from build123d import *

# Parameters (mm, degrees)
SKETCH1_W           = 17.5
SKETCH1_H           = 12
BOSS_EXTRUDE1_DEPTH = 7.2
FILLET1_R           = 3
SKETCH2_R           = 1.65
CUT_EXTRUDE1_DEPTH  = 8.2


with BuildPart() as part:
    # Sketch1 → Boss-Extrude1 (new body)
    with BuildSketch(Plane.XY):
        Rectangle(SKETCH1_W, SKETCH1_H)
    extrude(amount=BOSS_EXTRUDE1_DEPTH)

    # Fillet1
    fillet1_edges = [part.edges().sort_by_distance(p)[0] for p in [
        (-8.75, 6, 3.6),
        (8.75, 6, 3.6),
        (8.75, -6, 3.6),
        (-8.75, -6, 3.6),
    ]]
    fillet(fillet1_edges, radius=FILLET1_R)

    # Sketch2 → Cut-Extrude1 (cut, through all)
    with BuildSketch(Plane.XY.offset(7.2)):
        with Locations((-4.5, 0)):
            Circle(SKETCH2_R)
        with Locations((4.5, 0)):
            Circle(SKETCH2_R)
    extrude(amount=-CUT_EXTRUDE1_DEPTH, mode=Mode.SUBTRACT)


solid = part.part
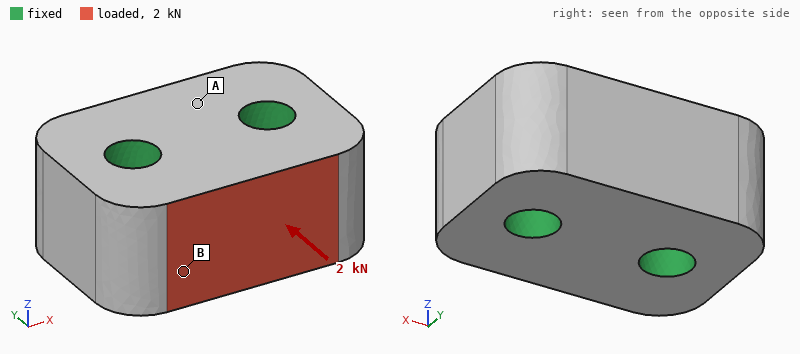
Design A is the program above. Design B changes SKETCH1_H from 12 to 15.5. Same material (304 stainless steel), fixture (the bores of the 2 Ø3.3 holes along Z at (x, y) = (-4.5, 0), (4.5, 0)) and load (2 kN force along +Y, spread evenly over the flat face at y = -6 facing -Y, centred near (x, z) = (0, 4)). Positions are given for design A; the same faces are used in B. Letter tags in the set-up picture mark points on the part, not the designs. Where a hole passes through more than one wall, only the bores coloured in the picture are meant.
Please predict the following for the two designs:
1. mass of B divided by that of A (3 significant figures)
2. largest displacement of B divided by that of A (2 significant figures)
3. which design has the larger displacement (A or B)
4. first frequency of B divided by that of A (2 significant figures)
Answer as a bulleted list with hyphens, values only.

- 1.33
- 1.2
- B
- 0.68
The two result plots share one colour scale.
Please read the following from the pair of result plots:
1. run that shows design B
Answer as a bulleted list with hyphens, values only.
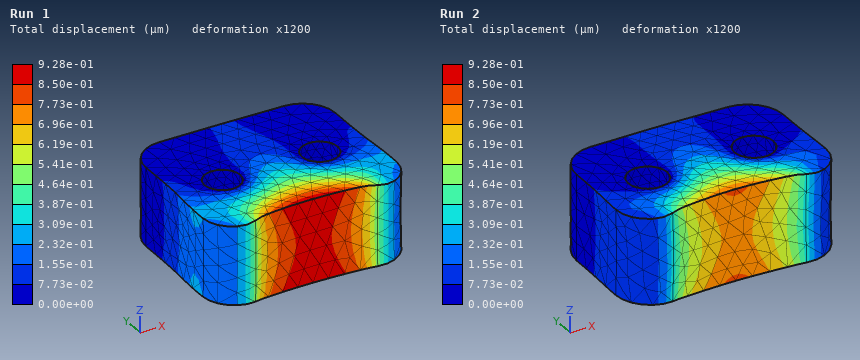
- Run 1
